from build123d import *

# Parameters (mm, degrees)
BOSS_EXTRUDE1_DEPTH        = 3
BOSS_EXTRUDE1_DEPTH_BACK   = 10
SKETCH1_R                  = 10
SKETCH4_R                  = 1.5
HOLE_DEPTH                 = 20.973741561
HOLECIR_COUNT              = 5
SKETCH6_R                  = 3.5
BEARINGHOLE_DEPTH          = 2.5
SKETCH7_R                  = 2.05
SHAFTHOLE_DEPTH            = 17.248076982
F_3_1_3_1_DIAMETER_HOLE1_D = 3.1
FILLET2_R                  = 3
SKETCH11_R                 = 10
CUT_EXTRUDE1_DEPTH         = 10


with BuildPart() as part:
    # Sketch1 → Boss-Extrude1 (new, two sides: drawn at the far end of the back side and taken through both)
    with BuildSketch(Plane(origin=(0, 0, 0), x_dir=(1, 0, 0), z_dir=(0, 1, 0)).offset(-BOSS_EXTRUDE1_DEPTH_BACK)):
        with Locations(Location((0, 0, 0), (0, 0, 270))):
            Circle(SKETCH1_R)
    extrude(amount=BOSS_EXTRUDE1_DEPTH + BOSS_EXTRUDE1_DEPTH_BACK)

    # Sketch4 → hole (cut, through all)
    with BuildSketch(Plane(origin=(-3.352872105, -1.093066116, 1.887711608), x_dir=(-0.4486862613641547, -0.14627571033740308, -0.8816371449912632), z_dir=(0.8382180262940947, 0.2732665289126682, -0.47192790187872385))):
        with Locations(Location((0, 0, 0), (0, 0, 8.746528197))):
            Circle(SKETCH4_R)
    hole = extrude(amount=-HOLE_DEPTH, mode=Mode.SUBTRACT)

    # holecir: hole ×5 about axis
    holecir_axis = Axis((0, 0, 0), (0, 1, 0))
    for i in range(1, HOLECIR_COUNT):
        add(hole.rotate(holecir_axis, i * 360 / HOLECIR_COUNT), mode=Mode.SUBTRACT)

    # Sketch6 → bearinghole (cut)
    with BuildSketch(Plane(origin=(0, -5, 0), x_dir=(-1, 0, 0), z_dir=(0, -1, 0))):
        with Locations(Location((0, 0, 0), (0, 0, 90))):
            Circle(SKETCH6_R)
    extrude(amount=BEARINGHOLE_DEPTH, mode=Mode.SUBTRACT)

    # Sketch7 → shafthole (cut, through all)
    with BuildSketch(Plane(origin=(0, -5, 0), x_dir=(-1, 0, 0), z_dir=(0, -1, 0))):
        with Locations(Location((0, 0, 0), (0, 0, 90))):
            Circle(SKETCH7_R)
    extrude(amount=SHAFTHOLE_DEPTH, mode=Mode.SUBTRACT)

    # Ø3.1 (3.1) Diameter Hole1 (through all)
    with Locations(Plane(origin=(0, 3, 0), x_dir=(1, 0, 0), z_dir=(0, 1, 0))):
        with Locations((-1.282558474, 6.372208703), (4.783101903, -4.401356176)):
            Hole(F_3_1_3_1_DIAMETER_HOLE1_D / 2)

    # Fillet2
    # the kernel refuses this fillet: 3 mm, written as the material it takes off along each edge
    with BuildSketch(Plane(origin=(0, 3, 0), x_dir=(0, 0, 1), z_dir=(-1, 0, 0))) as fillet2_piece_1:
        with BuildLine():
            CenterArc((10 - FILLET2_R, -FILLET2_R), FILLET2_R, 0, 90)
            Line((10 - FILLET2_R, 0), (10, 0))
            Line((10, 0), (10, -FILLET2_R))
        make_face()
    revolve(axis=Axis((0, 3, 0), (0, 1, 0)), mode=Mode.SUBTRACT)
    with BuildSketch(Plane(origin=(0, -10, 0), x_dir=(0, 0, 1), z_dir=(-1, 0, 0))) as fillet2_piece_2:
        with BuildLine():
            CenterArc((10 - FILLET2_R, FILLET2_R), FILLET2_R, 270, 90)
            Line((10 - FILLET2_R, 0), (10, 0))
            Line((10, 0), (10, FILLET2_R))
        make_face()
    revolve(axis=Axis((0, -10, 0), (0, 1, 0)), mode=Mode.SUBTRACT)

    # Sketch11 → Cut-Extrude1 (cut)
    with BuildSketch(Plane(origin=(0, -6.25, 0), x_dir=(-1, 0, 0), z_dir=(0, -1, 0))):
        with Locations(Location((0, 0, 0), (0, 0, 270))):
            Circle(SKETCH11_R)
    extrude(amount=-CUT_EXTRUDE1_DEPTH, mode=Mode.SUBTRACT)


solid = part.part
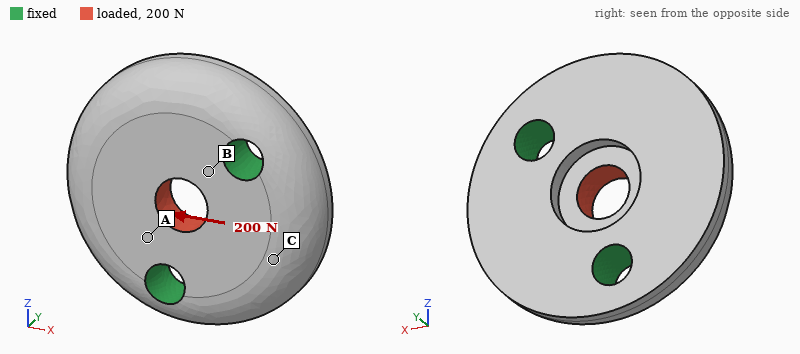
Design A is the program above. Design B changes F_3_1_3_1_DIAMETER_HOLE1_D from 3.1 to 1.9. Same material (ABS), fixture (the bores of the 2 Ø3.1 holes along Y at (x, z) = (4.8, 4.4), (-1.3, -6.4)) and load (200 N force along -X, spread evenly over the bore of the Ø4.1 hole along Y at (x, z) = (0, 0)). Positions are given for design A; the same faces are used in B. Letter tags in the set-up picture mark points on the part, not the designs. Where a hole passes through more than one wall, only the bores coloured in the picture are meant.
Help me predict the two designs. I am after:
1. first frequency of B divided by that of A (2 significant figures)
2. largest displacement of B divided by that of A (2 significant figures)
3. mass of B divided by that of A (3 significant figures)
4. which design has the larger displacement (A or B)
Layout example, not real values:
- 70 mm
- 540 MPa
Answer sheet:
- 0.86
- 1.3
- 1.04
- B
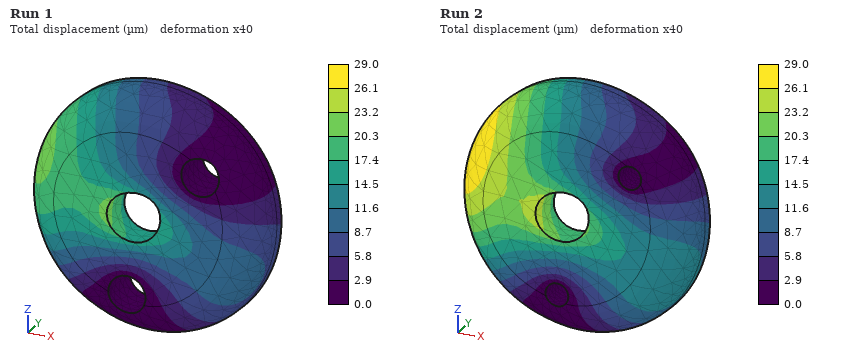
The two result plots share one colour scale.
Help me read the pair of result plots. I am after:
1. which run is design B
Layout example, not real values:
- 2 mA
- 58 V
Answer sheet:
- Run 2
